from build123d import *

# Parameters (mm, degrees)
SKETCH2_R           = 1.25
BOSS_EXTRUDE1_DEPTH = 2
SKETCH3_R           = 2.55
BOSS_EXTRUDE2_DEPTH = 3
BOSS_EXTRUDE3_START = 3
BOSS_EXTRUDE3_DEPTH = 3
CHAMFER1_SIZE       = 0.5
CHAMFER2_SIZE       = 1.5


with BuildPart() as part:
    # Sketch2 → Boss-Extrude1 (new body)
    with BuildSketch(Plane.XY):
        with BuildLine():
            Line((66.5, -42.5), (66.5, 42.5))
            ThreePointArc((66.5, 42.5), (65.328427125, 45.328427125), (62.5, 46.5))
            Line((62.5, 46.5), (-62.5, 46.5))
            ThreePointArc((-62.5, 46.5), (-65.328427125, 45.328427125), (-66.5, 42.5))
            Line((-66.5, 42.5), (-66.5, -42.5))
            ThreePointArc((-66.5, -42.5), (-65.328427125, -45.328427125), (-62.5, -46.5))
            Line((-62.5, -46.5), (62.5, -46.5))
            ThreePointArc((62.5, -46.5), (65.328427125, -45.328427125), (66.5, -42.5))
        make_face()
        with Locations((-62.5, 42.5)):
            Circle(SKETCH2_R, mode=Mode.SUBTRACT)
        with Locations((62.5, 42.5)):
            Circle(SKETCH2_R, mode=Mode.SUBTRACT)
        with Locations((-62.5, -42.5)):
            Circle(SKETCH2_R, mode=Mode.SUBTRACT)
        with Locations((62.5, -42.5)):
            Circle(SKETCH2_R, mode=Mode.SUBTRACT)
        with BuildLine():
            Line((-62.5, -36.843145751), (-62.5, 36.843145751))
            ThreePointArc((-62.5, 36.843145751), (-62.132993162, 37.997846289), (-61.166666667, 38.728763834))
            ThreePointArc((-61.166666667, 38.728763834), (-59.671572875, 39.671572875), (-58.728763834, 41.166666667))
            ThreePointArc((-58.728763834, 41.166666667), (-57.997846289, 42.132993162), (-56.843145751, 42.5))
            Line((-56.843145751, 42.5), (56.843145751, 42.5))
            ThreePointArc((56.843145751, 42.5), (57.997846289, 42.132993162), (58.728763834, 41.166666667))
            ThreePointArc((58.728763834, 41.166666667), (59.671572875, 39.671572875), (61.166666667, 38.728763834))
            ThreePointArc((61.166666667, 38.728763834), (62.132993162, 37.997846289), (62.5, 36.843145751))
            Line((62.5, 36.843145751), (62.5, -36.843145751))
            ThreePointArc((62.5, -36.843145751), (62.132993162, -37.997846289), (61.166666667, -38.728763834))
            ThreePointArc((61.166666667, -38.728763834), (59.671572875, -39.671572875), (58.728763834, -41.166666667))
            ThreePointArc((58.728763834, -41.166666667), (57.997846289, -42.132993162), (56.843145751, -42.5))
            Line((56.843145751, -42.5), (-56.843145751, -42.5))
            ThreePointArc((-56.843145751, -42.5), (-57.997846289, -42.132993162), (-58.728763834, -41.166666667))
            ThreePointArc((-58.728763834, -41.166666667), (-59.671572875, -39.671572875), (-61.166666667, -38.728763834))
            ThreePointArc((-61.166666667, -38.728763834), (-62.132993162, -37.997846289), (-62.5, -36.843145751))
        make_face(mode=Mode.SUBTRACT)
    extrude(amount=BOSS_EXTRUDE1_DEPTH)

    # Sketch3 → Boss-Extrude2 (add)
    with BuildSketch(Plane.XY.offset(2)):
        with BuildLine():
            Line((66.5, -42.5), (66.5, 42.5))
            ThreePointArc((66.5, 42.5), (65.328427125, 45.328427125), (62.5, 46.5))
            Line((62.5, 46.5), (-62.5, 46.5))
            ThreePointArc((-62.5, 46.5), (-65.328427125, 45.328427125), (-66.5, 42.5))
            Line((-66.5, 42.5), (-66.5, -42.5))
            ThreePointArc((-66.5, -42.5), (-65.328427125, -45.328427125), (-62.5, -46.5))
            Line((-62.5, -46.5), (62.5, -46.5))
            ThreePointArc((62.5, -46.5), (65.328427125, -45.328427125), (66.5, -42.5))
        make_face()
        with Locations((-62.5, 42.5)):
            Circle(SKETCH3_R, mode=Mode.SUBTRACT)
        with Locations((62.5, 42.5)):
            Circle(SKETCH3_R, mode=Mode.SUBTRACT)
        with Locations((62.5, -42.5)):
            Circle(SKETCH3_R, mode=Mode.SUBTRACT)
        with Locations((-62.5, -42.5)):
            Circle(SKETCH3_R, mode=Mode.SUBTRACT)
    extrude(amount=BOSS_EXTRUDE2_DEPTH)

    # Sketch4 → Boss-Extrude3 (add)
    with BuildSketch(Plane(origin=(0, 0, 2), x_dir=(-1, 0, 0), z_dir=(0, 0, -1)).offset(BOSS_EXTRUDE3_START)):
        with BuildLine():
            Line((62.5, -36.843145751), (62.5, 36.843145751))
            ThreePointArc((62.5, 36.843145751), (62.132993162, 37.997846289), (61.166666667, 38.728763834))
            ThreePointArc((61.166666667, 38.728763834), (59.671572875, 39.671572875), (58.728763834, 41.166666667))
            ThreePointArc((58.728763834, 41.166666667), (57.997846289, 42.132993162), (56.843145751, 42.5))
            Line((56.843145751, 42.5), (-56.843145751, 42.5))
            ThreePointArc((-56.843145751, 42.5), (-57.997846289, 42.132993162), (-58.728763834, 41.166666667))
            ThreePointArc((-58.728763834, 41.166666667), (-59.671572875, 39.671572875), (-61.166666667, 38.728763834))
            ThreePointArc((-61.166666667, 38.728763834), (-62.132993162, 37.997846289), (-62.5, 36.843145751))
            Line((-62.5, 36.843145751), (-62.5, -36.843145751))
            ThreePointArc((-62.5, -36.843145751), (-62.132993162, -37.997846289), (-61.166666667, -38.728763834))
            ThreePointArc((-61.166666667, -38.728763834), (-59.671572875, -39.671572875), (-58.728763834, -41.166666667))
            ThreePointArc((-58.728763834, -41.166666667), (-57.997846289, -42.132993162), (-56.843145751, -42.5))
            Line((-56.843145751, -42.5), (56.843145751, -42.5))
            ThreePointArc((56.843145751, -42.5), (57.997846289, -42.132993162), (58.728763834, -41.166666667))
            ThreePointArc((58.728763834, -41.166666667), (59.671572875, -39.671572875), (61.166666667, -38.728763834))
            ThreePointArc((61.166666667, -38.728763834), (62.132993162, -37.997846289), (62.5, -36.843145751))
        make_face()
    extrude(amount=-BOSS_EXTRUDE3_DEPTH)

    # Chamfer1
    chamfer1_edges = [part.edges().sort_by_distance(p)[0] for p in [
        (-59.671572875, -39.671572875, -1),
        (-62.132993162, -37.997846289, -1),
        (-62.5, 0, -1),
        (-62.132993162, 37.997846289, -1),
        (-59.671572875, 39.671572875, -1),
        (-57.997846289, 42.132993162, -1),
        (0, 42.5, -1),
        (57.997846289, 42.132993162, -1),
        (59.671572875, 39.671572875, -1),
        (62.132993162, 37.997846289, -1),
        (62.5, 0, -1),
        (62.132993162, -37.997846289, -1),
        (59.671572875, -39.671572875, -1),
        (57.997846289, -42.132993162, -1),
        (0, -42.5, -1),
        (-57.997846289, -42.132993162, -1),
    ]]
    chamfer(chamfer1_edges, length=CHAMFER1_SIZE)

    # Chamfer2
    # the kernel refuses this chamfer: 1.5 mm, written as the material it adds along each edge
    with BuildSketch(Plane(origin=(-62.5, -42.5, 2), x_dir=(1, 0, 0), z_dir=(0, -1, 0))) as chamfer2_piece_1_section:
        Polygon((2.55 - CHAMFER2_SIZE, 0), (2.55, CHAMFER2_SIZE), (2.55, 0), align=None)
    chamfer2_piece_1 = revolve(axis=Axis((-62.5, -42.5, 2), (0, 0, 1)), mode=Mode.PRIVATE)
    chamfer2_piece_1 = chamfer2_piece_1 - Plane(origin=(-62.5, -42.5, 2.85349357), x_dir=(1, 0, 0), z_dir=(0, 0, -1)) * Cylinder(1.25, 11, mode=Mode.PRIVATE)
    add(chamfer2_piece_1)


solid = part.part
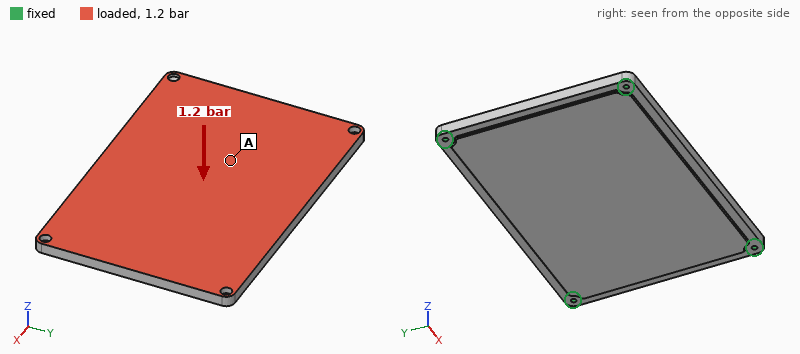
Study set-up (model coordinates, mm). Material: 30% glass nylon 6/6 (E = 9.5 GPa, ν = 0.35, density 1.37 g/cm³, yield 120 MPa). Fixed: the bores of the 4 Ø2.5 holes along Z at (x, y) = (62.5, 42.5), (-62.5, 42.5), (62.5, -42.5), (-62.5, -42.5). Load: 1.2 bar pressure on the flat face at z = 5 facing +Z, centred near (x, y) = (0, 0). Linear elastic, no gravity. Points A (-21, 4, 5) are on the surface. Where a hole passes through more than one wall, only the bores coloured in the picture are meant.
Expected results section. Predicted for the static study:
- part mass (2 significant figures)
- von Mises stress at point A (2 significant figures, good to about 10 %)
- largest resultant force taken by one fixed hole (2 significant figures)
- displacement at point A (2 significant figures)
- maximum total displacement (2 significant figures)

99 g
21 MPa
710 N
1.5 mm
1.6 mm
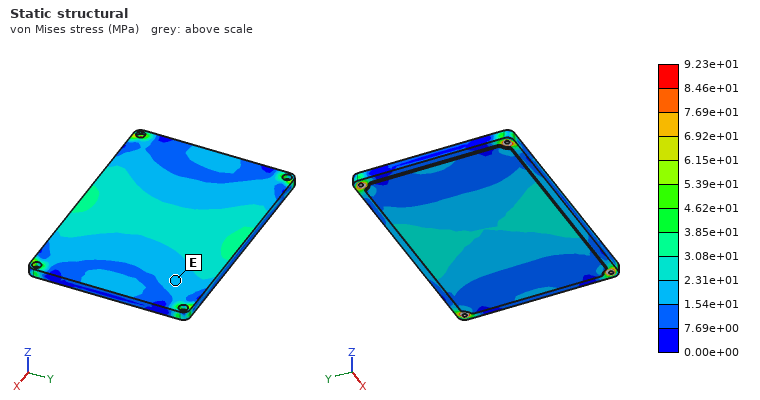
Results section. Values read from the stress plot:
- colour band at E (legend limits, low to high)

1.54e+01 to 2.31e+01 MPa
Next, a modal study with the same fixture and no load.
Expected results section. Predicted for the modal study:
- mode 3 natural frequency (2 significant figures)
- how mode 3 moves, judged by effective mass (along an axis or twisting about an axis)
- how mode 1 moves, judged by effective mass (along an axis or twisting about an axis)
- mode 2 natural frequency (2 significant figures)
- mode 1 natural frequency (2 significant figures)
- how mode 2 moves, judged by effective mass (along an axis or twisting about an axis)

1400 Hz
twisting about Y
along Z
1100 Hz
540 Hz
twisting about X
